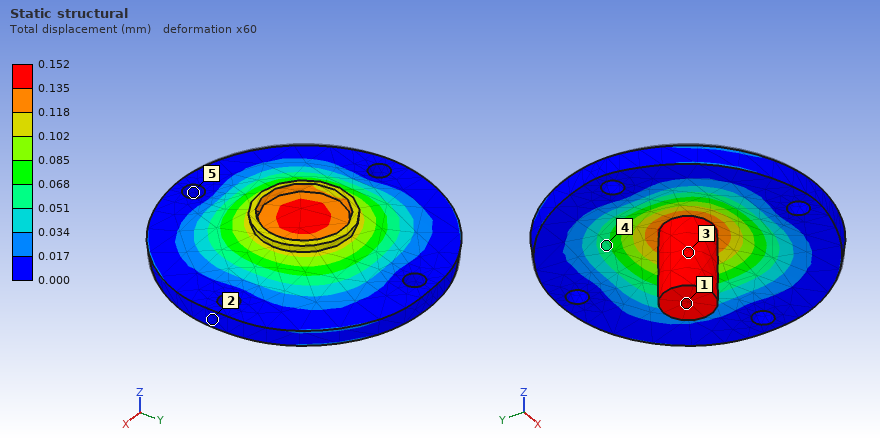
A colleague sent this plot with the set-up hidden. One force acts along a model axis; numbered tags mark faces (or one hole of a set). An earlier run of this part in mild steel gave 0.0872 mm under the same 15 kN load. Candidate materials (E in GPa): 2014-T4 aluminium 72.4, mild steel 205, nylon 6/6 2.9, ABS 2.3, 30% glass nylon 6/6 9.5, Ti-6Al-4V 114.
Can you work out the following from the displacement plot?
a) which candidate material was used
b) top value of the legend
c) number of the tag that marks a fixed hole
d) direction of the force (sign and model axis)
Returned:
Ti-6Al-4V
0.152 mm
5
+Z
